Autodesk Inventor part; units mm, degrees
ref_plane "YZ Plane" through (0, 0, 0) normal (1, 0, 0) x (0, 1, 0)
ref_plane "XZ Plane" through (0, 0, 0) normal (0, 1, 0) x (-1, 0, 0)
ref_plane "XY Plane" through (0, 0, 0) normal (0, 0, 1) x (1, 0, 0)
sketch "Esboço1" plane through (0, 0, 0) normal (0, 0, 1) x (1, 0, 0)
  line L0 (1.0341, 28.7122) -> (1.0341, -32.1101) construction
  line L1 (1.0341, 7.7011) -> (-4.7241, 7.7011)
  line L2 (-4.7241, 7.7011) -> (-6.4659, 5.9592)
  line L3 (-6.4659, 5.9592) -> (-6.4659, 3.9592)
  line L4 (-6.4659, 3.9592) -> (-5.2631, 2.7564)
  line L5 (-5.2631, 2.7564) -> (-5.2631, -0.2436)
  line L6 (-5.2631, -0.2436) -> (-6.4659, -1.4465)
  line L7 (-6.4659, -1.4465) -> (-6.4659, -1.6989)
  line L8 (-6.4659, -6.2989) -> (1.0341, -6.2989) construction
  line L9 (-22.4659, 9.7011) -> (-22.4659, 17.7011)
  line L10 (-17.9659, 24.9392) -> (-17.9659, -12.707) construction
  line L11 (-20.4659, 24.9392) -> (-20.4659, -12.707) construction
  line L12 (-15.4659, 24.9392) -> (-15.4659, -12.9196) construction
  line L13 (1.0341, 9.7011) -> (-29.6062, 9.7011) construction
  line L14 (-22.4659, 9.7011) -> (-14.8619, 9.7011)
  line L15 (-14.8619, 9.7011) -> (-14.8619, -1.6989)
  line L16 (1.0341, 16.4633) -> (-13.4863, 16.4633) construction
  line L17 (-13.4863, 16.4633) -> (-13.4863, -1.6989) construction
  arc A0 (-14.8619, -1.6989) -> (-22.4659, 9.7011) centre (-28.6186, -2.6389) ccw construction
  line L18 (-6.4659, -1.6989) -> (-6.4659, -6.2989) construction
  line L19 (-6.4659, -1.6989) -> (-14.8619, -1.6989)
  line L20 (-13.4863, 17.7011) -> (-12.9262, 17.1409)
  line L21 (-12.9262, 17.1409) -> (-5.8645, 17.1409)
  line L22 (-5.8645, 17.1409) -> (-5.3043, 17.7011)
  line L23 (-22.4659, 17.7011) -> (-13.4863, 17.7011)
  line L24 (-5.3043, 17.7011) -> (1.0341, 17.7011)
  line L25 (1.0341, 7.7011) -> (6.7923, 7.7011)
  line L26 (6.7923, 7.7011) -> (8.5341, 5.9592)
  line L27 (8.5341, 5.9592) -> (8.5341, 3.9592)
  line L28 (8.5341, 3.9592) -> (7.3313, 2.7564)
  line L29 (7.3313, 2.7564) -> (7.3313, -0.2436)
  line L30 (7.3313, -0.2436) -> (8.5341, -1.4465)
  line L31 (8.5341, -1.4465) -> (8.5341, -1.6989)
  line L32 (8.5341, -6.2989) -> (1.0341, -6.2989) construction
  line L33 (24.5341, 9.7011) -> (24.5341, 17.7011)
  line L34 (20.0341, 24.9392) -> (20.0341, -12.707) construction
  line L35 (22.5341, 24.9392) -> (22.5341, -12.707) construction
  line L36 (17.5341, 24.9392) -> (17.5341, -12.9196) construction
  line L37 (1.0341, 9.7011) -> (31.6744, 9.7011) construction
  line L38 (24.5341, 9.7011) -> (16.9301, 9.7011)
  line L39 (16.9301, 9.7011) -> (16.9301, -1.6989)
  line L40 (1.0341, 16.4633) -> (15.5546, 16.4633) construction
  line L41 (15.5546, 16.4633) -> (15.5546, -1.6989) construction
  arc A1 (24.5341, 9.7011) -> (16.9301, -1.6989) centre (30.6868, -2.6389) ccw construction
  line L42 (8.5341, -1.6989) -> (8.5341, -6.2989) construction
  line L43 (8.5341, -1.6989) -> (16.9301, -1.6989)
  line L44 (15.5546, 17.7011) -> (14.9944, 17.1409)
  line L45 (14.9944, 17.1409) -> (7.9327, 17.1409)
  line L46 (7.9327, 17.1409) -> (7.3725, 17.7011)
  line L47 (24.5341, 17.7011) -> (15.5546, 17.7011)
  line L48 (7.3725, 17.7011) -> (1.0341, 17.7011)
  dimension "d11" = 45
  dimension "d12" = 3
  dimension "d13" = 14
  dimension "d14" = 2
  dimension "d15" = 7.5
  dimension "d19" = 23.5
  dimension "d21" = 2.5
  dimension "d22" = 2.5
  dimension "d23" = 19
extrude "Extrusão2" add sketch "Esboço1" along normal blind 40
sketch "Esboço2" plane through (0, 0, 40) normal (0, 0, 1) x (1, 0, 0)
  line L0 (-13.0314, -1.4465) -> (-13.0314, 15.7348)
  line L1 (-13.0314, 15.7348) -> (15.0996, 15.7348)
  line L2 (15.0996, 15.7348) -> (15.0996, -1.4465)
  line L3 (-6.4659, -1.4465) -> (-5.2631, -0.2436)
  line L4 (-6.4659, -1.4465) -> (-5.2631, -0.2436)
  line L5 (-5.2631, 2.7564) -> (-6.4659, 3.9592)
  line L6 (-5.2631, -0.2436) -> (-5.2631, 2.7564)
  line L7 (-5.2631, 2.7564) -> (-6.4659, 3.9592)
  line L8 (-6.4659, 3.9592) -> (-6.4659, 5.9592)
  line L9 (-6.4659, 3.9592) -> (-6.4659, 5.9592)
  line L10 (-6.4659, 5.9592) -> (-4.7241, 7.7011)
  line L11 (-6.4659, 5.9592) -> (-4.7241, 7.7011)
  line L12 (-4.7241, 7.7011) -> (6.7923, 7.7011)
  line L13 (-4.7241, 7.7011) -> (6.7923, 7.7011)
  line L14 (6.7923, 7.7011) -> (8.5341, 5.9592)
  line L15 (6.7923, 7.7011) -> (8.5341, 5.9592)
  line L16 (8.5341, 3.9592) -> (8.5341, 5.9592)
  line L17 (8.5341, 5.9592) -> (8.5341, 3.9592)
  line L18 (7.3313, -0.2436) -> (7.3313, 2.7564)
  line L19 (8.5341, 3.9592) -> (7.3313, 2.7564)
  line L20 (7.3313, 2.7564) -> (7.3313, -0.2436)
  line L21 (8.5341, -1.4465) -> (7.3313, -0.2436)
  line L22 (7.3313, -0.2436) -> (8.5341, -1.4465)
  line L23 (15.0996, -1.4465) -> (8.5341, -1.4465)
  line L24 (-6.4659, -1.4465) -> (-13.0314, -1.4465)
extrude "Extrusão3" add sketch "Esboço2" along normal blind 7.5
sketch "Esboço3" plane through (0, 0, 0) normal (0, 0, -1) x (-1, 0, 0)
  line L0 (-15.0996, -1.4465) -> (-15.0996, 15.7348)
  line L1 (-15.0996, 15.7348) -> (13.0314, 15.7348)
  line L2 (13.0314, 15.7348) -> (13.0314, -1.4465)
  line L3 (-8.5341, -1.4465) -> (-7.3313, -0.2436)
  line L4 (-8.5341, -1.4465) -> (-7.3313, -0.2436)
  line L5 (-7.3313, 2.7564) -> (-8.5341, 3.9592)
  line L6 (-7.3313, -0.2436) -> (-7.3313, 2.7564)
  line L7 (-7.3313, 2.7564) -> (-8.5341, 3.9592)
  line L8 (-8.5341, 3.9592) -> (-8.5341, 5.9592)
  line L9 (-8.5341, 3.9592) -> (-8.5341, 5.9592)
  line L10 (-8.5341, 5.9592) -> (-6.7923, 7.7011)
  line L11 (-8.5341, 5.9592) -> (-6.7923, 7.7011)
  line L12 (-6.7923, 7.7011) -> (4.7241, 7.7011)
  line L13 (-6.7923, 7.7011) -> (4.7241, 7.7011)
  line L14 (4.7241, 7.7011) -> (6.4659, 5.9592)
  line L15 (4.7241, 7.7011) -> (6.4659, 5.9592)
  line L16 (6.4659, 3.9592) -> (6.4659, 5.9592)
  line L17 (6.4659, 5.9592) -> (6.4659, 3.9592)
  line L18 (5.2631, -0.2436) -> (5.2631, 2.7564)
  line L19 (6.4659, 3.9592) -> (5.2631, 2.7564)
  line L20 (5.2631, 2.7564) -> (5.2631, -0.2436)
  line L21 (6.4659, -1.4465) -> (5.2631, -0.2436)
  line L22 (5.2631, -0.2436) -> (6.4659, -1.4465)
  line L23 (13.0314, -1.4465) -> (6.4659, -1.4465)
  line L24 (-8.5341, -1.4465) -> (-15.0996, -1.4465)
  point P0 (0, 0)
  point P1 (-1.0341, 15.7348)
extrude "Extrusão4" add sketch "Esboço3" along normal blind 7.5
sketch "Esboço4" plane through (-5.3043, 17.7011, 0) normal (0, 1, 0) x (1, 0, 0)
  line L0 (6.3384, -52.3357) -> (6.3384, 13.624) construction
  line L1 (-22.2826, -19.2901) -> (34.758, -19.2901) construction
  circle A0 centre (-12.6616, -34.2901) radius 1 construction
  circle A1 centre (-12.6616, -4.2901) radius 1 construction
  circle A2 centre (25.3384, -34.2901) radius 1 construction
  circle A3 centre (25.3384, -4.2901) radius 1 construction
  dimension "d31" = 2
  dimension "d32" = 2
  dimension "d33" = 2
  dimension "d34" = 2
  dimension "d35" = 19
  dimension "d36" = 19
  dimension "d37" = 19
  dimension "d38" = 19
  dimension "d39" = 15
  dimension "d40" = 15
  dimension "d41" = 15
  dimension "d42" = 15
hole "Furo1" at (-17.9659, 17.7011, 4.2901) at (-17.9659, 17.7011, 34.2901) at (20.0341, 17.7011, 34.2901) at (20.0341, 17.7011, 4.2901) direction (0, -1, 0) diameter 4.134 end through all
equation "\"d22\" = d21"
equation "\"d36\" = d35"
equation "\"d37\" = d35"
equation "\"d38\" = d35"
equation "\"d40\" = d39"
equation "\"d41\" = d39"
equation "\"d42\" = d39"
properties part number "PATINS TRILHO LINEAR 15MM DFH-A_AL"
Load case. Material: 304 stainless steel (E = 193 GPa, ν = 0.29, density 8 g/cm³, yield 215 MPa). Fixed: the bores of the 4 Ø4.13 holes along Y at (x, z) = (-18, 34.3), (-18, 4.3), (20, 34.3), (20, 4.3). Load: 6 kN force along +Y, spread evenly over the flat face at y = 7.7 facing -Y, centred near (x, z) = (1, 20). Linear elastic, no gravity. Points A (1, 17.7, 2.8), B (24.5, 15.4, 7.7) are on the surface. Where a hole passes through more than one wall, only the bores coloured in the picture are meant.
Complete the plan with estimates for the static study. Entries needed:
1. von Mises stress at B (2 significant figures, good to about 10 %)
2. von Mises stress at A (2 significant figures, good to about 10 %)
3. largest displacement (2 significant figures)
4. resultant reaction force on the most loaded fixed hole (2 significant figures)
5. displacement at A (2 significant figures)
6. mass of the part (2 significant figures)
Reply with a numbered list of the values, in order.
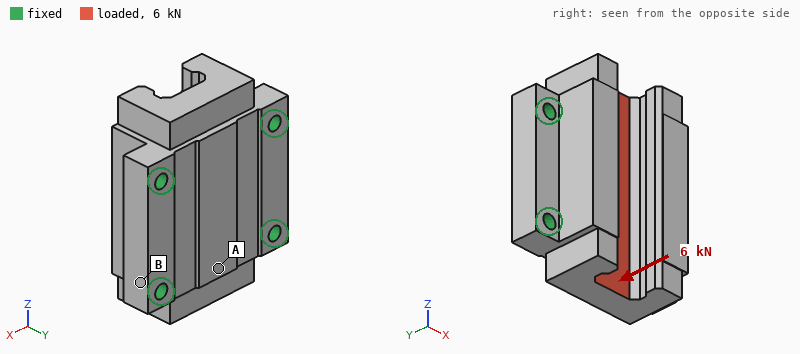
1. 14 MPa
2. 34 MPa
3. 6.6 µm
4. 1.7 kN
5. 5.1 µm
6. 230 g
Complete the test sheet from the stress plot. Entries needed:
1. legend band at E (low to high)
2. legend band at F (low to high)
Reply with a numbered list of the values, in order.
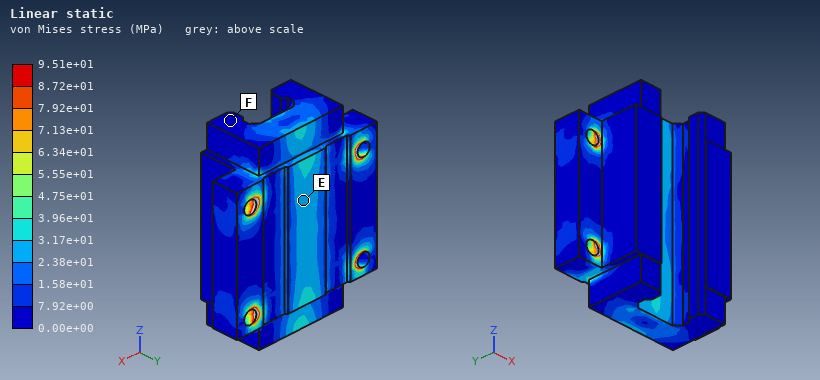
1. 2.38e+01 to 3.17e+01 MPa
2. 0.00e+00 to 7.92e+00 MPa
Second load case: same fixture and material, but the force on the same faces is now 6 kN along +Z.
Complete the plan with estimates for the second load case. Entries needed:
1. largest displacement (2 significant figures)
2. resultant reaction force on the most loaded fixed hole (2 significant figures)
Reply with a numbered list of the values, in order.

1. 4.3 µm
2. 1.7 kN
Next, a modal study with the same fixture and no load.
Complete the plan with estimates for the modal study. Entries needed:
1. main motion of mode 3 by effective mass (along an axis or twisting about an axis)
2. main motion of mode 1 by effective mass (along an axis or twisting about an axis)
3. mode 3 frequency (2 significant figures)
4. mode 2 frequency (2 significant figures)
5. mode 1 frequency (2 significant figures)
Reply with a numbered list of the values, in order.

1. along Z
2. along Y
3. 25 kHz
4. 16 kHz
5. 15 kHz
